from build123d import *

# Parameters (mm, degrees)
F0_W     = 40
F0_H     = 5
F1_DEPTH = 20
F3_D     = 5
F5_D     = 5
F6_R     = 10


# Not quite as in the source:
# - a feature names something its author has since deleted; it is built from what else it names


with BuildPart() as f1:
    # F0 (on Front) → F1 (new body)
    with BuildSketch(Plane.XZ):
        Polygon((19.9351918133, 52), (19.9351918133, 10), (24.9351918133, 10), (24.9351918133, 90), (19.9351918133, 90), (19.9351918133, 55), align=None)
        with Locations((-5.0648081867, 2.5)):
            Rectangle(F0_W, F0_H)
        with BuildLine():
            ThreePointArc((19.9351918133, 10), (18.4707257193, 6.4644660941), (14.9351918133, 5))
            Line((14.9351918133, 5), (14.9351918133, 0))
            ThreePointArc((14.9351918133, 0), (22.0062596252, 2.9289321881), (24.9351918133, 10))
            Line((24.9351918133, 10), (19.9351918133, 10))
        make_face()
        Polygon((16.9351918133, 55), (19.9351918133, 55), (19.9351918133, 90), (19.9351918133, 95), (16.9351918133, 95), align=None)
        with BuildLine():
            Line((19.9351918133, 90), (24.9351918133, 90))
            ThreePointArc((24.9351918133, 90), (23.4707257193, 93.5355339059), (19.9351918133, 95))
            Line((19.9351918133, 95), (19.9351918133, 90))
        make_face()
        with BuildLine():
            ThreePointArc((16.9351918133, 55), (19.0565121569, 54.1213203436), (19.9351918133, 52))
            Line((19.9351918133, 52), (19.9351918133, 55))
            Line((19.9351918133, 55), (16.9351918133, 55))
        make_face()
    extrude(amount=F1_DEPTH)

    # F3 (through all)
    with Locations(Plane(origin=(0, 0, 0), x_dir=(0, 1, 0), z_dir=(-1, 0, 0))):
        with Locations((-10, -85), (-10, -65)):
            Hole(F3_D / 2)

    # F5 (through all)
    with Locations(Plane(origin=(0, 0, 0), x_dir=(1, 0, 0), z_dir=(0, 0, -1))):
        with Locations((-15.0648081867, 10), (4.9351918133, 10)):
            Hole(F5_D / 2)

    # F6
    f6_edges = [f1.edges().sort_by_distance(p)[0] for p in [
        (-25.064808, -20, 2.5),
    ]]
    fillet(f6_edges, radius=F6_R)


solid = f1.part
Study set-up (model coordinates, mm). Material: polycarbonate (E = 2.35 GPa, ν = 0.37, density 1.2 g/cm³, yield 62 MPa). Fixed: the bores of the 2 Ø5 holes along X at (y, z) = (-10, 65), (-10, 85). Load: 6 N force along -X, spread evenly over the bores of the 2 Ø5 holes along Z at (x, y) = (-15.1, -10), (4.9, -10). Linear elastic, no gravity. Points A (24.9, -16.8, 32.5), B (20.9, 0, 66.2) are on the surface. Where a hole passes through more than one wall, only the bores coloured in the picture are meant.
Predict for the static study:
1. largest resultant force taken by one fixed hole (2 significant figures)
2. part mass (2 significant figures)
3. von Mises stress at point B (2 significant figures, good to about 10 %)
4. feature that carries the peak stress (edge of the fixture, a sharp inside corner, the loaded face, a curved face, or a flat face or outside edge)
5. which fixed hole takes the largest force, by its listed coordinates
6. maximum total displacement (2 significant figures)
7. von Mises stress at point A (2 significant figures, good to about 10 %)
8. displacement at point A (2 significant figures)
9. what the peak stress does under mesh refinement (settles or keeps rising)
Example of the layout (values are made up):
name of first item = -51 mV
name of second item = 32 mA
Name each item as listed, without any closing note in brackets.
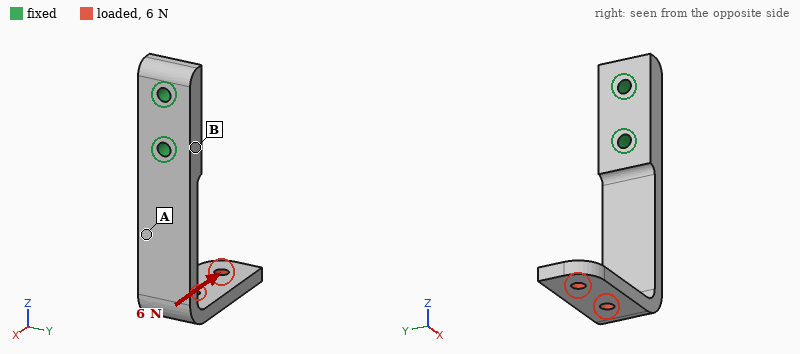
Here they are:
largest resultant force taken by one fixed hole = 10 N
part mass = 18 g
von Mises stress at point B = 0.50 MPa
feature that carries the peak stress = edge of the fixture
which fixed hole takes the largest force, by its listed coordinates = (-10, 65)
maximum total displacement = 1.1 mm
von Mises stress at point A = 2.2 MPa
displacement at point A = 0.19 mm
what the peak stress does under mesh refinement = keeps rising
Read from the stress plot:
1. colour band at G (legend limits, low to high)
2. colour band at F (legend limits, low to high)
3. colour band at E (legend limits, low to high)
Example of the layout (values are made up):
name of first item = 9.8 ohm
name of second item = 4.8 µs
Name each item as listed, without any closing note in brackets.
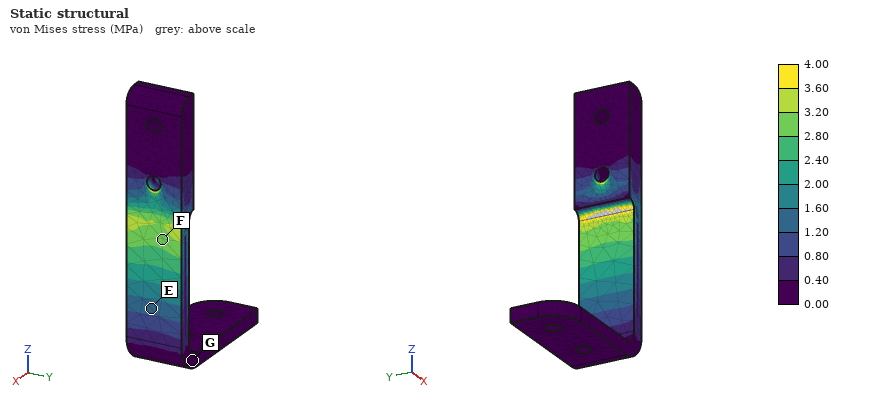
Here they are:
colour band at G = 0.00 to 0.40 MPa
colour band at F = 2.80 to 3.20 MPa
colour band at E = 1.20 to 1.60 MPa
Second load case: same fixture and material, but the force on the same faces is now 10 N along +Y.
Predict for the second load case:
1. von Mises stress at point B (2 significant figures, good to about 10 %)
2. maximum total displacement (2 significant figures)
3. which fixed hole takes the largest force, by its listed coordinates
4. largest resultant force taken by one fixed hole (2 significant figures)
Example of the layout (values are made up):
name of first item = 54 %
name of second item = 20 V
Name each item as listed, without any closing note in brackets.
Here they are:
von Mises stress at point B = 0.93 MPa
maximum total displacement = 1.2 mm
which fixed hole takes the largest force, by its listed coordinates = (-10, 65)
largest resultant force taken by one fixed hole = 29 N
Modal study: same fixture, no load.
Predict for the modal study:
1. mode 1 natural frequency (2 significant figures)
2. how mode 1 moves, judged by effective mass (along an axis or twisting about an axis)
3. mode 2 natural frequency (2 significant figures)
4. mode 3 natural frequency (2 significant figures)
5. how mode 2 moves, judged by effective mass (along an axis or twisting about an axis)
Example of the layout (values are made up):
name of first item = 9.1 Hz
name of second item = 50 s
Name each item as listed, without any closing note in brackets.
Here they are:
mode 1 natural frequency = 150 Hz
how mode 1 moves, judged by effective mass = along X
mode 2 natural frequency = 250 Hz
mode 3 natural frequency = 440 Hz
how mode 2 moves, judged by effective mass = along Y
